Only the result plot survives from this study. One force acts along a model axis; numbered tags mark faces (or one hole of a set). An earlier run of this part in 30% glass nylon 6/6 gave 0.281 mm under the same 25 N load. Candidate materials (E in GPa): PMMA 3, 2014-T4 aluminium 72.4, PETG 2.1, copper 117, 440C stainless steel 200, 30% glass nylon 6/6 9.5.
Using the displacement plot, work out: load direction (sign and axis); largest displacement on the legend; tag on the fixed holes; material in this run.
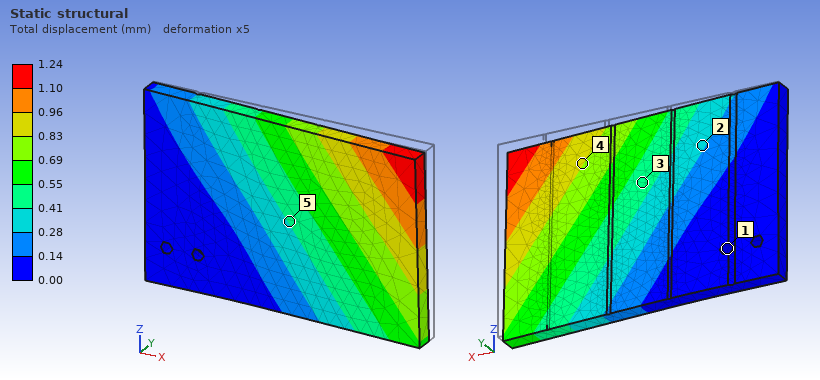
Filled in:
-Y
1.24 mm
1
PETG
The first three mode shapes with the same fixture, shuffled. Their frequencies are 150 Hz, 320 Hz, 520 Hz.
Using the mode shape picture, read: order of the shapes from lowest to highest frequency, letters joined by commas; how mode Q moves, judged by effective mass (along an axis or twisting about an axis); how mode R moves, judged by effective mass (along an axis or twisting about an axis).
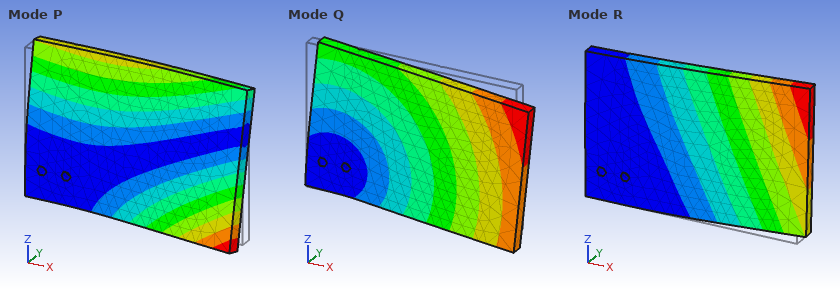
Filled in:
R, P, Q
along Z
along Y
